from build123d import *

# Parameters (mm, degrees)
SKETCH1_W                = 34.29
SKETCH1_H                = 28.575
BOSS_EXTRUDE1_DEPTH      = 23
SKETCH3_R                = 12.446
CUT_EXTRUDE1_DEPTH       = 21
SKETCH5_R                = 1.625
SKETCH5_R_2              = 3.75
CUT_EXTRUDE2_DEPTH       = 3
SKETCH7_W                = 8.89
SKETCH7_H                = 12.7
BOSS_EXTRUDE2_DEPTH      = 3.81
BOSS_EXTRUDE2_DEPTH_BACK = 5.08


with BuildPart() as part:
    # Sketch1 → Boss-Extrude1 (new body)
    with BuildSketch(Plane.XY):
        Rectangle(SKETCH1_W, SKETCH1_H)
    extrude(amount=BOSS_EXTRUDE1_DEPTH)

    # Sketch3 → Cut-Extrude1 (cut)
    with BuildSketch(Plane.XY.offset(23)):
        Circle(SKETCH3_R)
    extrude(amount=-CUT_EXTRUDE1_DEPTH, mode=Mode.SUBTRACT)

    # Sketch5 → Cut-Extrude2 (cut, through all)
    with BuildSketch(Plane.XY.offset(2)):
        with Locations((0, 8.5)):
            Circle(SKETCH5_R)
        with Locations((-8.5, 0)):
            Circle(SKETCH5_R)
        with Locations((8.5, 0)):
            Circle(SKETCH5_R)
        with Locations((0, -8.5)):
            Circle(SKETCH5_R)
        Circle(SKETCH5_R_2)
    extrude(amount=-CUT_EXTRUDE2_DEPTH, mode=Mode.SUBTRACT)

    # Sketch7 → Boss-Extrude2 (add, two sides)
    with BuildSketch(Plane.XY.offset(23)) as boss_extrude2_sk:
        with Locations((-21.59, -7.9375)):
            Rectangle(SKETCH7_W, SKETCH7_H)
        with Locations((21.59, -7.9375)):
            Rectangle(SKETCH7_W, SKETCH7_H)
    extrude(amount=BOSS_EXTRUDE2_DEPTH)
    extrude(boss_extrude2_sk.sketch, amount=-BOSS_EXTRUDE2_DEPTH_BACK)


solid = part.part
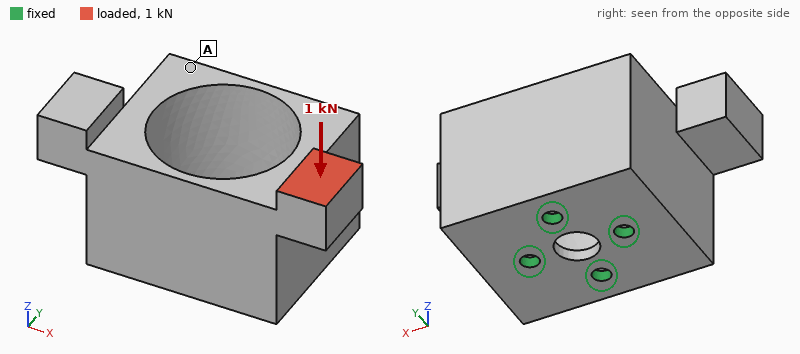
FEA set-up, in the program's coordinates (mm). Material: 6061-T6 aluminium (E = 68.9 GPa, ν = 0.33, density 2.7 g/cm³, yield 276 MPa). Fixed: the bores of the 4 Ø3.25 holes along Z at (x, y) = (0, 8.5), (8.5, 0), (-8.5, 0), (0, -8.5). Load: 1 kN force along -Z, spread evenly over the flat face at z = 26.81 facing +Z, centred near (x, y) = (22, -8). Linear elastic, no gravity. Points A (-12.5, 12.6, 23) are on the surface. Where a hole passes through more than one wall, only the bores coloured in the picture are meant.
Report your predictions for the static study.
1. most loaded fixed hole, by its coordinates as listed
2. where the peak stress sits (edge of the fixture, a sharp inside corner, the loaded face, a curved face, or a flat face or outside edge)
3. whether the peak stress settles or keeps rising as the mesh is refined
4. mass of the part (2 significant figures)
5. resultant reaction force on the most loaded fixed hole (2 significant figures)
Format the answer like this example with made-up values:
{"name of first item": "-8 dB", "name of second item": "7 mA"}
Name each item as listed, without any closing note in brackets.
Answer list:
{"most loaded fixed hole, by its coordinates as listed": "(8.5, 0)", "where the peak stress sits": "edge of the fixture", "whether the peak stress settles or keeps rising as the mesh is refined": "keeps rising", "mass of the part": "38 g", "resultant reaction force on the most loaded fixed hole": "1.3 kN"}
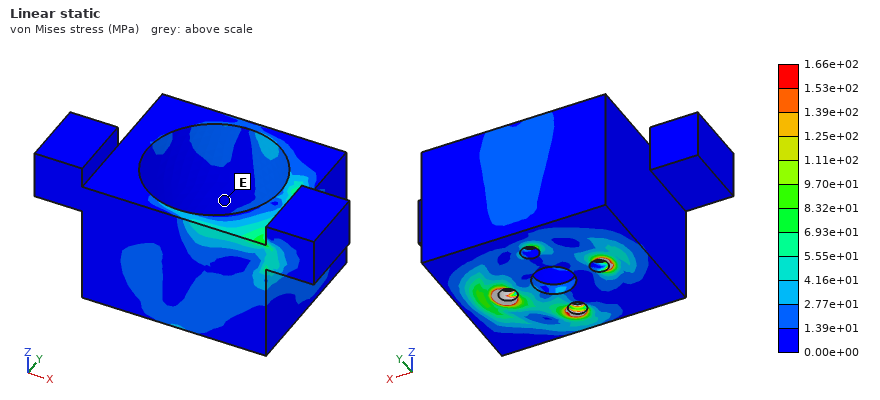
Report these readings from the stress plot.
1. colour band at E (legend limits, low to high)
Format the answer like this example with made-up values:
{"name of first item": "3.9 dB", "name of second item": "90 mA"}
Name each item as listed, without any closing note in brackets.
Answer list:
{"colour band at E": "0.00e+00 to 1.39e+01 MPa"}
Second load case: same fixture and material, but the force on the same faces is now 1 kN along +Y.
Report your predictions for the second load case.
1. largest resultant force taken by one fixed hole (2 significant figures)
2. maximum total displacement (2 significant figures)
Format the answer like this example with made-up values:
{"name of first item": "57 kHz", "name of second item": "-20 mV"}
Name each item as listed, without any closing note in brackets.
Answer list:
{"largest resultant force taken by one fixed hole": "1.3 kN", "maximum total displacement": "0.13 mm"}
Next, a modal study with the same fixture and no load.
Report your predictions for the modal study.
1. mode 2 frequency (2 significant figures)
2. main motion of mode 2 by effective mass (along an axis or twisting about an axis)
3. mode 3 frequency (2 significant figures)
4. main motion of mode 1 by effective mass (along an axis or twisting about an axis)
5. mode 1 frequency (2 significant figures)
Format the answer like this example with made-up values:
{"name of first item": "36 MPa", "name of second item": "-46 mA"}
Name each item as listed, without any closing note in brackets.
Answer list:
{"mode 2 frequency": "4700 Hz", "main motion of mode 2 by effective mass": "along Y", "mode 3 frequency": "9600 Hz", "main motion of mode 1 by effective mass": "along X", "mode 1 frequency": "4300 Hz"}
